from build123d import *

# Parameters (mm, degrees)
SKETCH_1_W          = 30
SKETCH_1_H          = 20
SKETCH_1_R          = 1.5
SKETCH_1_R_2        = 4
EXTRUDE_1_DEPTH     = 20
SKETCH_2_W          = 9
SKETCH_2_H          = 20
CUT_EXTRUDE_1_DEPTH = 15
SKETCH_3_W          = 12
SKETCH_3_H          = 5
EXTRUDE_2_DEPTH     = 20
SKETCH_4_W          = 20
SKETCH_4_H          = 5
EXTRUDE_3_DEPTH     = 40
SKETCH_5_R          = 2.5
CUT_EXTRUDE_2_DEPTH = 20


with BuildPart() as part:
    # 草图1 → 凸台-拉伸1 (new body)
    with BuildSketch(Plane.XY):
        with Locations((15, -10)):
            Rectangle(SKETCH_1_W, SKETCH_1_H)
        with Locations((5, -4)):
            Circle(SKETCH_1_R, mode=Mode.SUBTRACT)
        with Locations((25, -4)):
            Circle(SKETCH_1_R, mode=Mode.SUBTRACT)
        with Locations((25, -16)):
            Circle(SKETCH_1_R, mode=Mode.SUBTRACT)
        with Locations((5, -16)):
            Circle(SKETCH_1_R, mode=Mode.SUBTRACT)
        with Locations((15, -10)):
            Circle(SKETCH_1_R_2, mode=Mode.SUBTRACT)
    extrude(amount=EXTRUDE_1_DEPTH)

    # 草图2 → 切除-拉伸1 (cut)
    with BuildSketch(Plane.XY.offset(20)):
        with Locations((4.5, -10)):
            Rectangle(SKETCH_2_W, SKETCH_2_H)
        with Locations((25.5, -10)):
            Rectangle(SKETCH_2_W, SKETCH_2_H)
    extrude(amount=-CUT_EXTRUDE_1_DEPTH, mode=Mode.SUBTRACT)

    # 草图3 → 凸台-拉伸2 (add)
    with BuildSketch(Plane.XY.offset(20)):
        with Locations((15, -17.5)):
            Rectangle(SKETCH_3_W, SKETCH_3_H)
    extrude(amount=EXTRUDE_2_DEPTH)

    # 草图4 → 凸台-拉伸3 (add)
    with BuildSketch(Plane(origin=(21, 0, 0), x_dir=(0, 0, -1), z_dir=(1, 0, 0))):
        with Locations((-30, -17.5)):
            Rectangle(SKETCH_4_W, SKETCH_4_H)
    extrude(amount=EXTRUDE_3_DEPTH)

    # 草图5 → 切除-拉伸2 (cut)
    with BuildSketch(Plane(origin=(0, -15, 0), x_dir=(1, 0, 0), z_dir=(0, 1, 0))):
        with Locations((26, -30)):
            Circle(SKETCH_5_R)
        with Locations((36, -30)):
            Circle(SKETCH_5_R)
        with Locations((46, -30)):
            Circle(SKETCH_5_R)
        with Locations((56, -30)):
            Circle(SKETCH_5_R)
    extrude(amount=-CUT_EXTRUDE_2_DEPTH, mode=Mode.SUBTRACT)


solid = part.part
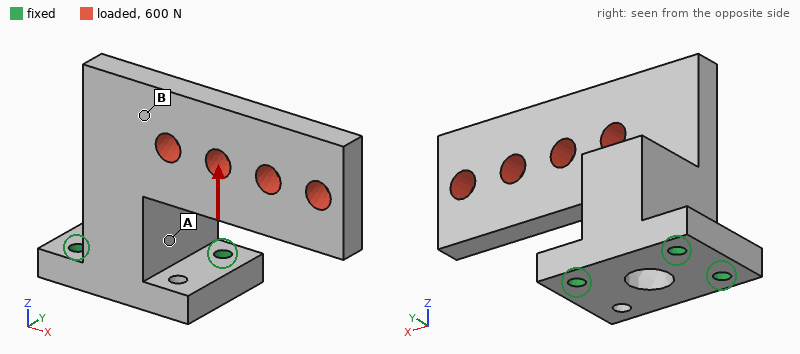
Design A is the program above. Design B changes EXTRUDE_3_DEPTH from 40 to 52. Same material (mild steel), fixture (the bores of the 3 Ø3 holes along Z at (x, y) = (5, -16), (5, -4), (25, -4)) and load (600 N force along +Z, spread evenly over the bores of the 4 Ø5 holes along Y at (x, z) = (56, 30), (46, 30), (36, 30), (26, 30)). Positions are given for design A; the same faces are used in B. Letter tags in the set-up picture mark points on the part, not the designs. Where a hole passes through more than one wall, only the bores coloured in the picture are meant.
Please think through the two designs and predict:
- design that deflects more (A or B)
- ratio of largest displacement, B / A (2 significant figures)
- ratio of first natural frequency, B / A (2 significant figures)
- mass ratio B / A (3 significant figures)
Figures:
B
1.2
0.65
1.12
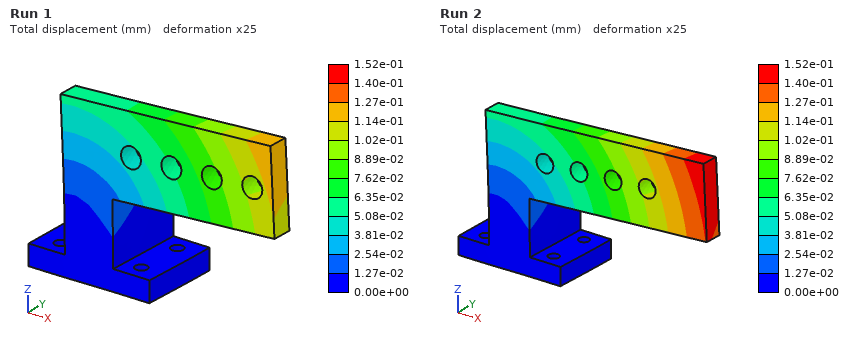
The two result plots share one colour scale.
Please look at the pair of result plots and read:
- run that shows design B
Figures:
Run 2
